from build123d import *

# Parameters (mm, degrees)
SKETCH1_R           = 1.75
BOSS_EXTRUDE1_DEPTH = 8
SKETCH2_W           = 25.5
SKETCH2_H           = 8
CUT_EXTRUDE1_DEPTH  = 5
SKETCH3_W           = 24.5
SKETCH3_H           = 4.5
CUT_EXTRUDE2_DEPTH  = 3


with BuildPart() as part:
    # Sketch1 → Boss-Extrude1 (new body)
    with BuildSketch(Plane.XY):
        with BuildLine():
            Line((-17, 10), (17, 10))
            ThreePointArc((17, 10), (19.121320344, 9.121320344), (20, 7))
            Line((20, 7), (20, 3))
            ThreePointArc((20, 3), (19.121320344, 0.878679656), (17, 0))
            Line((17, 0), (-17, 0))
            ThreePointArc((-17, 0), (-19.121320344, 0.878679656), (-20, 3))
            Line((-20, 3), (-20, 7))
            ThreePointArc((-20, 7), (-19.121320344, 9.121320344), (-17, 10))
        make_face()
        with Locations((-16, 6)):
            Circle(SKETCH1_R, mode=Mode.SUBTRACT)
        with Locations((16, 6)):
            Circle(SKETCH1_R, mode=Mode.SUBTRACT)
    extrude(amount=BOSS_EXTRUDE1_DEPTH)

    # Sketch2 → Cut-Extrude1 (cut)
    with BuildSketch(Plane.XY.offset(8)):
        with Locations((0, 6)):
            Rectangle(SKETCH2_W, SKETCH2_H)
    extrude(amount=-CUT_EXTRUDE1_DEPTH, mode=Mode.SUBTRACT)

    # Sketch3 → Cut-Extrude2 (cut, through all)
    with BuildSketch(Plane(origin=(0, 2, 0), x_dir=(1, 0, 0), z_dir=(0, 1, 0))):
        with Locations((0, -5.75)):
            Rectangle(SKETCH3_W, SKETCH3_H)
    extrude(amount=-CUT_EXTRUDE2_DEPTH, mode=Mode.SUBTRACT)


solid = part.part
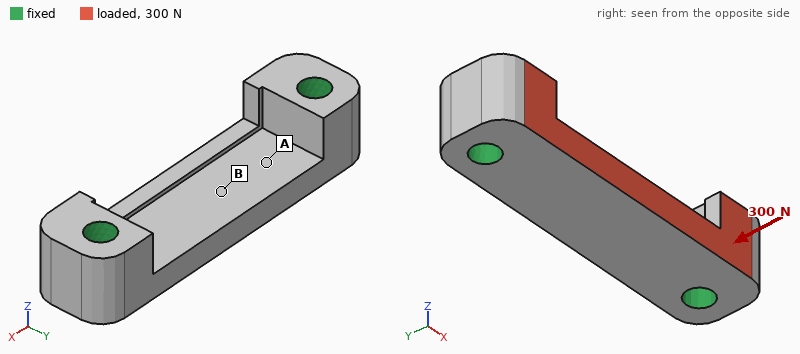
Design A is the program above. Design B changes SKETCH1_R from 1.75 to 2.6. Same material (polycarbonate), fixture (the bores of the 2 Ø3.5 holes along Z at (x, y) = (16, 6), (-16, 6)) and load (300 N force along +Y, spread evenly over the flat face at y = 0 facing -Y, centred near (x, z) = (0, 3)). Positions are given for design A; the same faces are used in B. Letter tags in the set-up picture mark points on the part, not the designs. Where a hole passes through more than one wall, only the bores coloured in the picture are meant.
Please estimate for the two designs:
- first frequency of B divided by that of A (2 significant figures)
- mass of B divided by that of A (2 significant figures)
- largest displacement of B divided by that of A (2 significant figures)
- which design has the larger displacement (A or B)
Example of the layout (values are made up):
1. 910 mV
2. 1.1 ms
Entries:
1. 1.1
2. 0.89
3. 0.84
4. A
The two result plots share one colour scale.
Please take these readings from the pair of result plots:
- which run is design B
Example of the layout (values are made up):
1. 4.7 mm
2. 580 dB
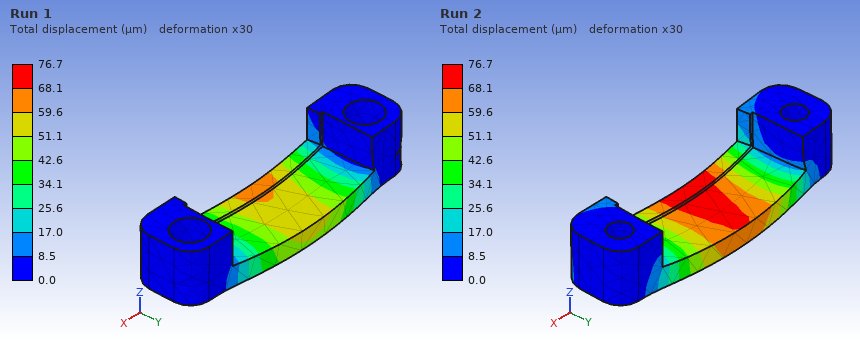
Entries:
1. Run 1
